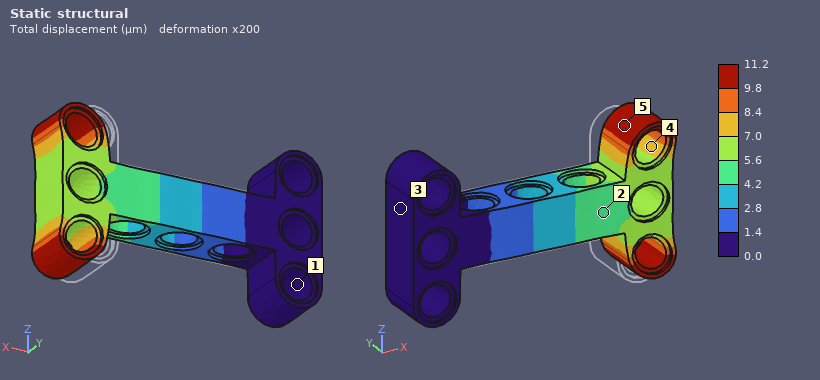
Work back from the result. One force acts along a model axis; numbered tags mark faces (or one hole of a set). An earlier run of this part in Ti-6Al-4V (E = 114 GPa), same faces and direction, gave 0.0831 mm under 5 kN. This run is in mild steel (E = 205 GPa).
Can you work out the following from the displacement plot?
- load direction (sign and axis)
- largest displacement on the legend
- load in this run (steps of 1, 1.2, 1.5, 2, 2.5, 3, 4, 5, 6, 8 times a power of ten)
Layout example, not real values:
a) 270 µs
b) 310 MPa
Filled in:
a) +X
b) 11.2 µm
c) 1.2 kN
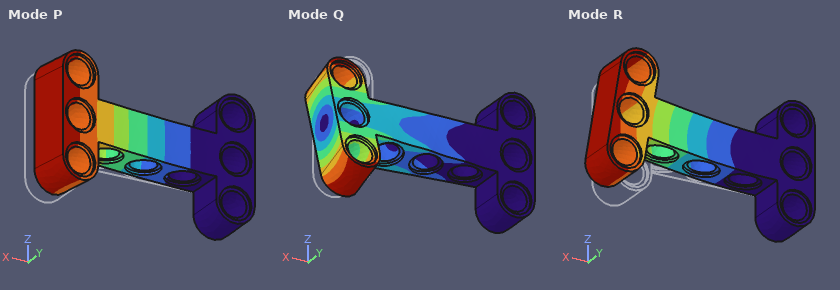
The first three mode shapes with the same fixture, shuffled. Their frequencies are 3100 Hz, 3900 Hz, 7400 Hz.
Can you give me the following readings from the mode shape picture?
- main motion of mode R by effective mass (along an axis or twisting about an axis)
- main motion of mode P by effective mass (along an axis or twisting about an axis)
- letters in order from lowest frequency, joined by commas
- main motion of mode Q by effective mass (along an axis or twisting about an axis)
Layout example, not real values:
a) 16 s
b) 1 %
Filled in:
a) along Z
b) along Y
c) R, P, Q
d) twisting about X
